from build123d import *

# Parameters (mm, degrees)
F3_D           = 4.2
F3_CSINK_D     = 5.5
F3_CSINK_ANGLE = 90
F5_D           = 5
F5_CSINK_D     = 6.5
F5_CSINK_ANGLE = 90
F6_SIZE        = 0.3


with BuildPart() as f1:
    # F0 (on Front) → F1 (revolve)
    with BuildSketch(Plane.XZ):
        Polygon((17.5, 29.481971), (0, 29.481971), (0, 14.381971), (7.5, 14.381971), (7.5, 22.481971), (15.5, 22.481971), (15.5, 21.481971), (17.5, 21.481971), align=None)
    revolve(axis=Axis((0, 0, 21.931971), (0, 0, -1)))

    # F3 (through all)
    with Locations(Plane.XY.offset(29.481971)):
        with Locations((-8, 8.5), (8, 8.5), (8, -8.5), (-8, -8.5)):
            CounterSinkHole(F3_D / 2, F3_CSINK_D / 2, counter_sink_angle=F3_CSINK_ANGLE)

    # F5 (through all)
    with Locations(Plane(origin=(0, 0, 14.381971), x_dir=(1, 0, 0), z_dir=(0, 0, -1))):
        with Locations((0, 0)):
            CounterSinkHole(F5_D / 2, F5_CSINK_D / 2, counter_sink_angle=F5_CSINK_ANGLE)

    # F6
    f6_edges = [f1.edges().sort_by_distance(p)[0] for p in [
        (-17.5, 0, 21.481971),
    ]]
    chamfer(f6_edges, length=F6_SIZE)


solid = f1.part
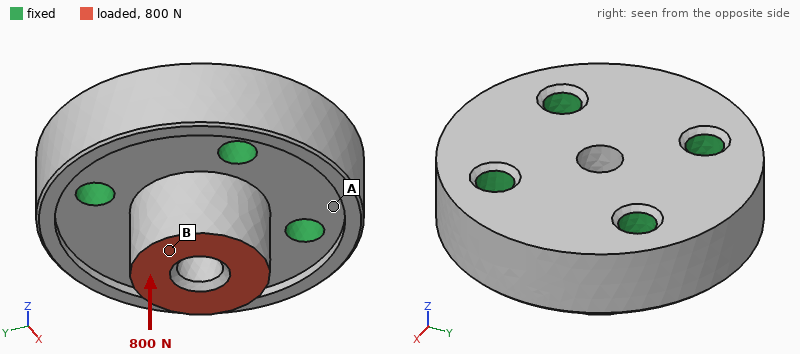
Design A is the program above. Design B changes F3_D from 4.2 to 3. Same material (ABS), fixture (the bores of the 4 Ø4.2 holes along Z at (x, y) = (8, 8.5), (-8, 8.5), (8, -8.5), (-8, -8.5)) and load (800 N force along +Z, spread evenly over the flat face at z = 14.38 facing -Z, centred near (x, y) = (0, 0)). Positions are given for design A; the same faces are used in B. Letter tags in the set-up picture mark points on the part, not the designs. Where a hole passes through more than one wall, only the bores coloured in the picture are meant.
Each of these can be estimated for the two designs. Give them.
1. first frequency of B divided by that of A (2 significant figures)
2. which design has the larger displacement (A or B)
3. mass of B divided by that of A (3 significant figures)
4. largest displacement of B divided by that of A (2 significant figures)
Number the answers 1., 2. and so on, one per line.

1. 0.87
2. B
3. 1.02
4. 1.1
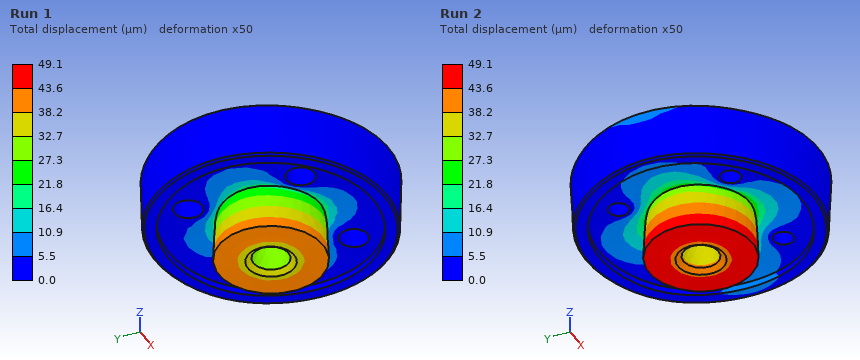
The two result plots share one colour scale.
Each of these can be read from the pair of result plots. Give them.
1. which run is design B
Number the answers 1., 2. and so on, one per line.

1. Run 2
